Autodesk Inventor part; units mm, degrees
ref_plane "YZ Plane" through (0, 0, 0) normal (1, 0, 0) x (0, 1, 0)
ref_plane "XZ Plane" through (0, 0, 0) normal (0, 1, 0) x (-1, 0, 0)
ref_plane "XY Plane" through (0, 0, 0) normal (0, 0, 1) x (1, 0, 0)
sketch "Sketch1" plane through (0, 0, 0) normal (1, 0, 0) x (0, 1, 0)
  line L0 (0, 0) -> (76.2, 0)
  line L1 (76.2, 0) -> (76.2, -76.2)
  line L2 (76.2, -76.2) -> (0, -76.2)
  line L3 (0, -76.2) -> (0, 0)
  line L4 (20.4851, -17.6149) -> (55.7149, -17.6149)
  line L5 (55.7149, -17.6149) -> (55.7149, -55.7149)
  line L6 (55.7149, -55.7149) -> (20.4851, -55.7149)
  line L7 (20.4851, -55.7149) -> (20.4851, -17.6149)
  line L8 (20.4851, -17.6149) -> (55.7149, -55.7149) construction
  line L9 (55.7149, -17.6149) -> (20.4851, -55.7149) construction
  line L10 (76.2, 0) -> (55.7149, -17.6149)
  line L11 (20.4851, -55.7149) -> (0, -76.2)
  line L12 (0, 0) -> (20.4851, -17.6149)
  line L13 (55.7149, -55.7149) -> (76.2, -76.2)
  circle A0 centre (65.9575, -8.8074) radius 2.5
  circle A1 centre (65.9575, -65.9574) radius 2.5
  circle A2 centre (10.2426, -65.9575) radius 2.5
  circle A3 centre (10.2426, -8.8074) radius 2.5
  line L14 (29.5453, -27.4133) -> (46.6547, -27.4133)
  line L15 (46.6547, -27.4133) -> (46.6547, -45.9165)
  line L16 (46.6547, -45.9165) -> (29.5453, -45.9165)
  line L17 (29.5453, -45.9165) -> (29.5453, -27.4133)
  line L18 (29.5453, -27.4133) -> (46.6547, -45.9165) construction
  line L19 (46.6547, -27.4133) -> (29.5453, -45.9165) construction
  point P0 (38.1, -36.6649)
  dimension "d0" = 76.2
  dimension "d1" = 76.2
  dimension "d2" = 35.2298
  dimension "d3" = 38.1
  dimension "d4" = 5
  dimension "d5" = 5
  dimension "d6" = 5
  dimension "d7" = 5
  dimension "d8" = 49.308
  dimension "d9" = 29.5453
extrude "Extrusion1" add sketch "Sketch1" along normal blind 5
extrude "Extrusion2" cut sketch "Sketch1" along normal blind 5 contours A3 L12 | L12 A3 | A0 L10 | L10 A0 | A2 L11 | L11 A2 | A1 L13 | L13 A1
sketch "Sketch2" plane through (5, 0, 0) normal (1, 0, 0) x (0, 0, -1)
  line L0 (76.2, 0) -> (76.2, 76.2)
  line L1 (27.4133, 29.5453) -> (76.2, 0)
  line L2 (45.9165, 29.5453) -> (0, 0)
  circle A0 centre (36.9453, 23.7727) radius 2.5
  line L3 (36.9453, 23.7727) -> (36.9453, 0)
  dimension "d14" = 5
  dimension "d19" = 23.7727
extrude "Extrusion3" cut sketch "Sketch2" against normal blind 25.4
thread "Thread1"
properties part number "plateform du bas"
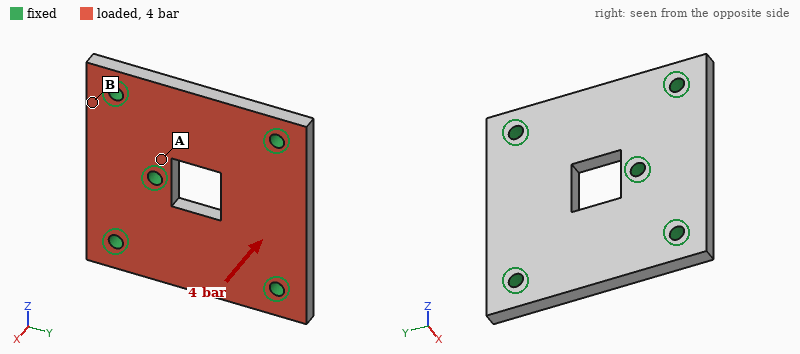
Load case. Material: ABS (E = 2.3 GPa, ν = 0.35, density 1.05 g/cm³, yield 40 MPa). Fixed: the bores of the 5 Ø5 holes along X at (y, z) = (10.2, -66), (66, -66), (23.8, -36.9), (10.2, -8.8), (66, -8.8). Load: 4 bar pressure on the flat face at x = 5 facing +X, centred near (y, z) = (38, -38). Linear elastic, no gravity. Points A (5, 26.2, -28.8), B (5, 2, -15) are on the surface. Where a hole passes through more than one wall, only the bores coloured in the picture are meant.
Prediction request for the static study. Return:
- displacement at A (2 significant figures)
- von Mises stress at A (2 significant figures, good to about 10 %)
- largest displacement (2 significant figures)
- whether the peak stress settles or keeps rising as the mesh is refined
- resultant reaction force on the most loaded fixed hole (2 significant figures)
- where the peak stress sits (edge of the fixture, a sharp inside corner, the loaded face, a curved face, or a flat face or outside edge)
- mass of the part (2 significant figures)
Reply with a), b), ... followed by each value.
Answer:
a) 0.10 mm
b) 13 MPa
c) 0.61 mm
d) keeps rising
e) 510 N
f) edge of the fixture
g) 28 g
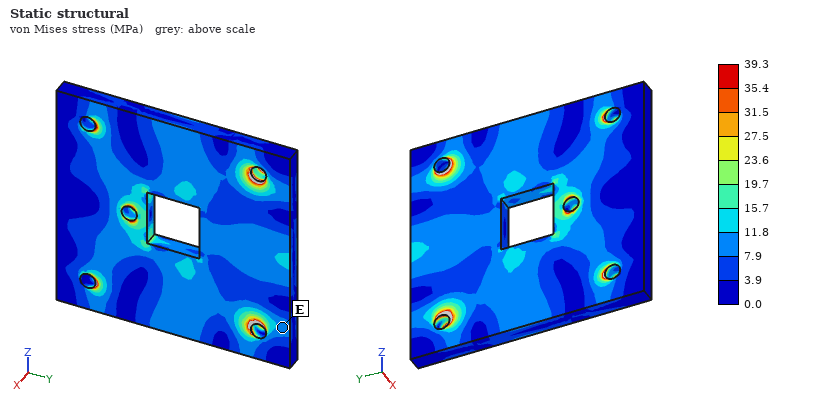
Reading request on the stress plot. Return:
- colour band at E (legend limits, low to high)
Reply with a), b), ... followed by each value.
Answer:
a) 7.9 to 11.8 MPa
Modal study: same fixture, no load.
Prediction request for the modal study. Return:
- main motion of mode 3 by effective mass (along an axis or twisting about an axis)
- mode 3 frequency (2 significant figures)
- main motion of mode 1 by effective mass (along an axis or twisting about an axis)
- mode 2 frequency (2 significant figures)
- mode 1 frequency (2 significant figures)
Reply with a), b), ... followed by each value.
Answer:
a) twisting about Y
b) 2700 Hz
c) along X
d) 2500 Hz
e) 2200 Hz
